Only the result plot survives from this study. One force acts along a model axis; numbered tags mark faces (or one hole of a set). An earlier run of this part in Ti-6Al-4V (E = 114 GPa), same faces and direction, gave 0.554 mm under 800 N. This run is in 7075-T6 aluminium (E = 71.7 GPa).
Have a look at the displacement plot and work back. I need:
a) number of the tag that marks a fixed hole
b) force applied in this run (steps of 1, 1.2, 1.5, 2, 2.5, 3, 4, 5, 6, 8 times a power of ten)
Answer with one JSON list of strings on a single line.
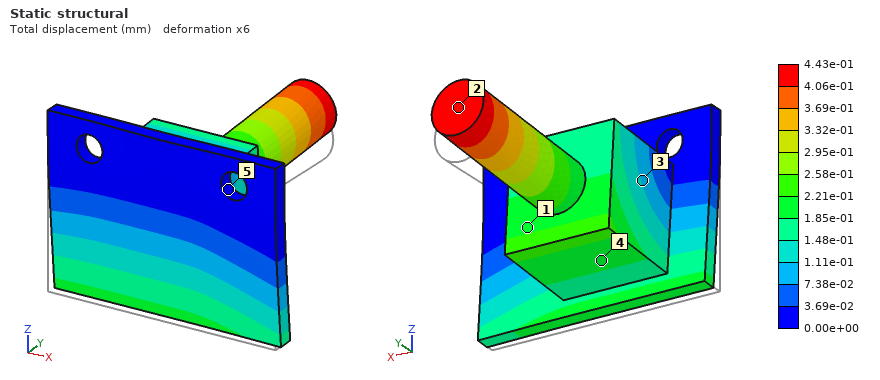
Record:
["5", "400 N"]
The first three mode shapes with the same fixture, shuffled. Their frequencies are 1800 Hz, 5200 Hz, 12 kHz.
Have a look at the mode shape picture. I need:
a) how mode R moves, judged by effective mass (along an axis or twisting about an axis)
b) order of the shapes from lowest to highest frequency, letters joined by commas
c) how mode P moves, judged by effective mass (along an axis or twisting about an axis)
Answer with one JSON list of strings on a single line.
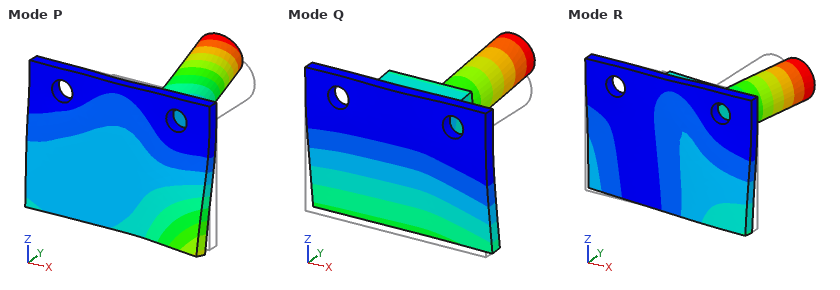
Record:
["along X", "Q, R, P", "along Y"]
